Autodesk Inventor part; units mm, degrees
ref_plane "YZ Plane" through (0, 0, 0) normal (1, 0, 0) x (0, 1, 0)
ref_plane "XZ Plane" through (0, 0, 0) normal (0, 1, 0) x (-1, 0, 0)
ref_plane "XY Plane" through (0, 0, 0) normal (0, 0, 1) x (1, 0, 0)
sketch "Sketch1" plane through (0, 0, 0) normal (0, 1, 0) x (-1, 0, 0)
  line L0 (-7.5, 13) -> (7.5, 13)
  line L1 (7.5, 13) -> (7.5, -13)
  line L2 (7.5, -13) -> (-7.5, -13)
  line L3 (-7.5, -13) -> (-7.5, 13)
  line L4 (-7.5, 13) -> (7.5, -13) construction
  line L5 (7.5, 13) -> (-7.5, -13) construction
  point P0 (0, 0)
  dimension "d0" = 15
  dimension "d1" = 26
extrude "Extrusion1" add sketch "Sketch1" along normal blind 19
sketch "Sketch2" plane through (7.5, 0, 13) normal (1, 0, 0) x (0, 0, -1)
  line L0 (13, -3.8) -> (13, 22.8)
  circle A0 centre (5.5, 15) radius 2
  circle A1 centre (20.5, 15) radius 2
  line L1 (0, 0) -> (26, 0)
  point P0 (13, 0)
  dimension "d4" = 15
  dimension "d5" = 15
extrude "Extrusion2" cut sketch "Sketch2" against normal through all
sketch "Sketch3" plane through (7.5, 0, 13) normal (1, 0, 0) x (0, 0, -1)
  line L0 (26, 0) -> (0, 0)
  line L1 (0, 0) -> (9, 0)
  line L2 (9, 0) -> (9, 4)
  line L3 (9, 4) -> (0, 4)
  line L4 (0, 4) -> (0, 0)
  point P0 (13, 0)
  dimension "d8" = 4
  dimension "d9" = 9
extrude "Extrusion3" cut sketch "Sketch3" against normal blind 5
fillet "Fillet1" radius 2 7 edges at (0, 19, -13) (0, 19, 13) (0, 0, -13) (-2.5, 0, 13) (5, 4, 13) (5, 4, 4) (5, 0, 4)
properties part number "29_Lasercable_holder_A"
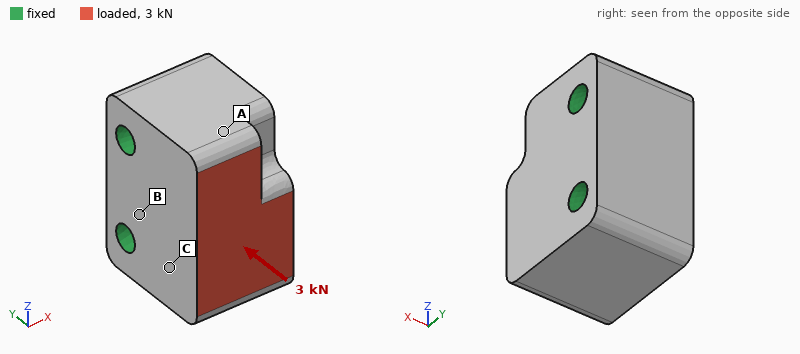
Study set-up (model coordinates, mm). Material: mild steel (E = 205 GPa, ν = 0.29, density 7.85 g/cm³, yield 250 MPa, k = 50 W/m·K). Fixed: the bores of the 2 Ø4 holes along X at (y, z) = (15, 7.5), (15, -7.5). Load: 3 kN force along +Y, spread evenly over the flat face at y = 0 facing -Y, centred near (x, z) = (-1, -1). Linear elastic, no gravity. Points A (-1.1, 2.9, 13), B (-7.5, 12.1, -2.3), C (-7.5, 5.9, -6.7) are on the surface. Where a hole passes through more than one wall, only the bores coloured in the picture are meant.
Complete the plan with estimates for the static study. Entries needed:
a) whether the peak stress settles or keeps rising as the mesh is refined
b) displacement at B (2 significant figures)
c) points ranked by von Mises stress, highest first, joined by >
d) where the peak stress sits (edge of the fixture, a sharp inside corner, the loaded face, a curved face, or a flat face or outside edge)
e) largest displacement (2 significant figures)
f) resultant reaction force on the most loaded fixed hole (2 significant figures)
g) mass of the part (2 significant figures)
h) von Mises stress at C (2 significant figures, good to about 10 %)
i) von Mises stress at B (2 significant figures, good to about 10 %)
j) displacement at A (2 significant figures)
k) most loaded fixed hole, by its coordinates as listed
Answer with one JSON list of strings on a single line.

["keeps rising", "0.32 µm", "C > B > A", "edge of the fixture", "0.92 µm", "1.7 kN", "53 g", "12 MPa", "6.8 MPa", "0.34 µm", "(15, -7.5)"]
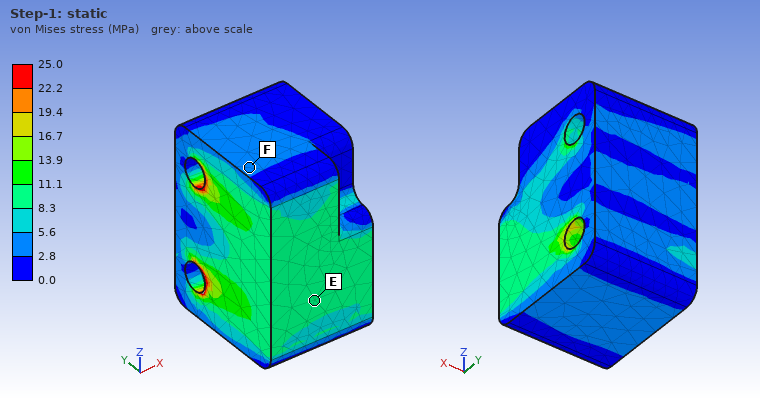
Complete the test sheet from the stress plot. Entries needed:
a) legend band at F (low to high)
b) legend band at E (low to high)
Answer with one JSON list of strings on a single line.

["2.8 to 5.6 MPa", "8.3 to 11.1 MPa"]
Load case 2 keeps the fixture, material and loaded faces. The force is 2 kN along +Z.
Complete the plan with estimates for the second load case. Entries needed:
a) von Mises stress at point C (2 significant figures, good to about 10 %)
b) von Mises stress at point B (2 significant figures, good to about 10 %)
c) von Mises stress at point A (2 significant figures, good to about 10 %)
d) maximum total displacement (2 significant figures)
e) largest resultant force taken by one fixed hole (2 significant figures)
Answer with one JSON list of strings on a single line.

["11 MPa", "11 MPa", "4.7 MPa", "2.0 µm", "1.9 kN"]
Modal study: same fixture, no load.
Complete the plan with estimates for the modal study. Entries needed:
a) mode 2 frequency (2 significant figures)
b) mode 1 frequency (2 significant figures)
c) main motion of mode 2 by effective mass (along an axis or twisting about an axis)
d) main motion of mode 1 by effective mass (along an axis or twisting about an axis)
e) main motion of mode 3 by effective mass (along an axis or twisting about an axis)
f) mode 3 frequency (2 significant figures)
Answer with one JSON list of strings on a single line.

["43 kHz", "36 kHz", "along Z", "along X", "twisting about Y", "51 kHz"]
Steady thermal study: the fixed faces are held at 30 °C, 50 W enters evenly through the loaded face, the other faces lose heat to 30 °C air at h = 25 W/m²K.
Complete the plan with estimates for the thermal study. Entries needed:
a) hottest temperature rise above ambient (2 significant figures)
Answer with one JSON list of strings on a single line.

["44 K"]
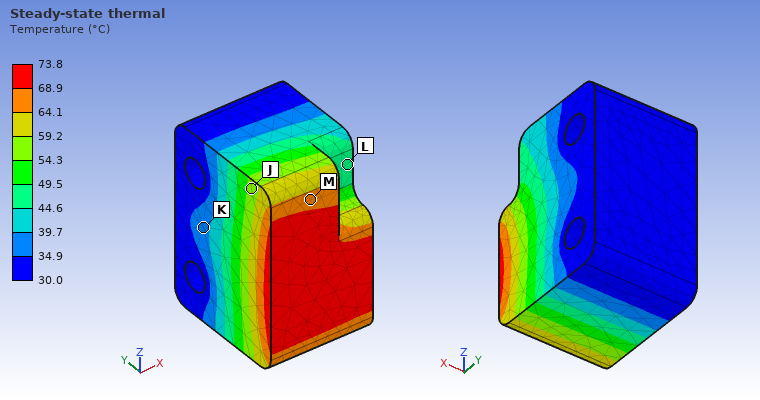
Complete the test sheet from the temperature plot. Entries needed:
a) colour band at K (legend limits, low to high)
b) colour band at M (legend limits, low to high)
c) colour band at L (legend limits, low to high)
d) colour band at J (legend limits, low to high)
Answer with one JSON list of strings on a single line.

["34.9 to 39.7 °C", "64.1 to 68.9 °C", "44.6 to 49.5 °C", "54.3 to 59.2 °C"]
